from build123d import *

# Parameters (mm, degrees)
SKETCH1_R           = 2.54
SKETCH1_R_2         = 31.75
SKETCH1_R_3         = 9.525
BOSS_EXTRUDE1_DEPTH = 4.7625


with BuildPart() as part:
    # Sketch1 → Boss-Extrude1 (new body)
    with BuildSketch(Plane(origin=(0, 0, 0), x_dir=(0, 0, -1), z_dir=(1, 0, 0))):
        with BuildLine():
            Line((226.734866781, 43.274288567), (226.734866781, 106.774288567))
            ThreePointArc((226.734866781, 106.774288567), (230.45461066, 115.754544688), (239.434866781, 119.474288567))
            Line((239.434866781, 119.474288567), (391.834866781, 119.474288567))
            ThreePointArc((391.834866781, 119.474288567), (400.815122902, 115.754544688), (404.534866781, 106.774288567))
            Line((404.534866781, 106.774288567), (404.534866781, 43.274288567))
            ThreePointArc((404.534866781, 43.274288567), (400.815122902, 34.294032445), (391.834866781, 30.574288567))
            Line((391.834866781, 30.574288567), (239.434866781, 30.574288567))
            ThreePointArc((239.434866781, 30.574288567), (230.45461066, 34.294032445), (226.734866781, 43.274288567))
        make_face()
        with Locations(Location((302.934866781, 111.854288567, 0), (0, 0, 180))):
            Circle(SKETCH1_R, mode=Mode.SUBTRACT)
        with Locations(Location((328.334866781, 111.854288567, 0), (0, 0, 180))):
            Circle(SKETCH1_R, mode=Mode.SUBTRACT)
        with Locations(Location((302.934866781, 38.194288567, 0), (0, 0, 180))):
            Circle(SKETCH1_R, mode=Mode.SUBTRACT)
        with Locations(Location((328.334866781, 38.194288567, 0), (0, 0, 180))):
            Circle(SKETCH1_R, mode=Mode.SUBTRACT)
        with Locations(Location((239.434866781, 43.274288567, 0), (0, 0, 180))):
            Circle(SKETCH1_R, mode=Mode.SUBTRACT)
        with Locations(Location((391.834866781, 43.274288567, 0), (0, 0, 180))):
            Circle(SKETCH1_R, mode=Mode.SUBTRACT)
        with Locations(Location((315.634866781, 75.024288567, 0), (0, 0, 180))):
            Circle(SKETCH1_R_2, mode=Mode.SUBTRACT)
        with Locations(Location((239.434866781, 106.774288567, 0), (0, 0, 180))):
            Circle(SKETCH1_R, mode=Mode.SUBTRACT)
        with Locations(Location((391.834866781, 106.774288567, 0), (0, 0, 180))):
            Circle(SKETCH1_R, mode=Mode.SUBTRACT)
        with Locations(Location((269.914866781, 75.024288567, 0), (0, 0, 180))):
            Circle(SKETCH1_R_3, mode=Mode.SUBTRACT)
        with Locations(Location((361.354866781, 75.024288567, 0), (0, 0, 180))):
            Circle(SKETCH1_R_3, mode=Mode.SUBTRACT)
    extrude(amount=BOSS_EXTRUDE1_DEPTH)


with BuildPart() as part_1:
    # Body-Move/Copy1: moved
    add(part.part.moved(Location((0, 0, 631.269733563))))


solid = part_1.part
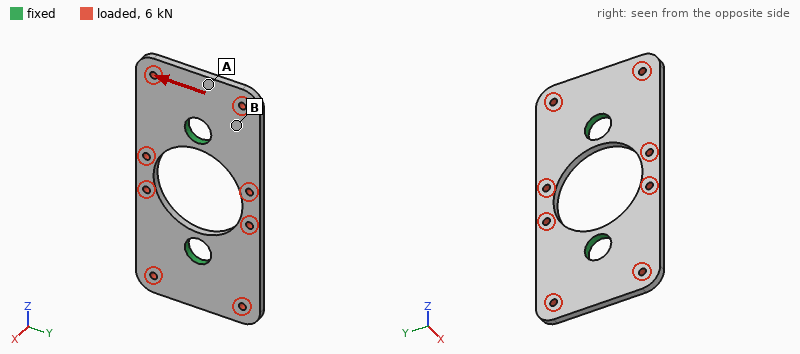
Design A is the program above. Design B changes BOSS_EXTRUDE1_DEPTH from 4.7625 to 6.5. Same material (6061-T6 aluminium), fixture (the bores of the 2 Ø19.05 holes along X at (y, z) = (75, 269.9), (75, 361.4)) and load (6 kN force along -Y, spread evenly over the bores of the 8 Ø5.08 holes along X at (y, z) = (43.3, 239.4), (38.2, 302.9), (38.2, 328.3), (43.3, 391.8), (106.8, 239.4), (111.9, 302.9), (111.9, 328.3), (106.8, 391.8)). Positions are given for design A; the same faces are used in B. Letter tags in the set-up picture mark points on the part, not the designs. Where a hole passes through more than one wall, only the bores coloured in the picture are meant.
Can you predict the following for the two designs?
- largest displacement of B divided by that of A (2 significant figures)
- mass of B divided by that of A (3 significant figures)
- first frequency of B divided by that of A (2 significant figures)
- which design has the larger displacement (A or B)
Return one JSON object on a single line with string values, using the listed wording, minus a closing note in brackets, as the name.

{"largest displacement of B divided by that of A": "0.73", "mass of B divided by that of A": "1.36", "first frequency of B divided by that of A": "1.3", "which design has the larger displacement": "A"}
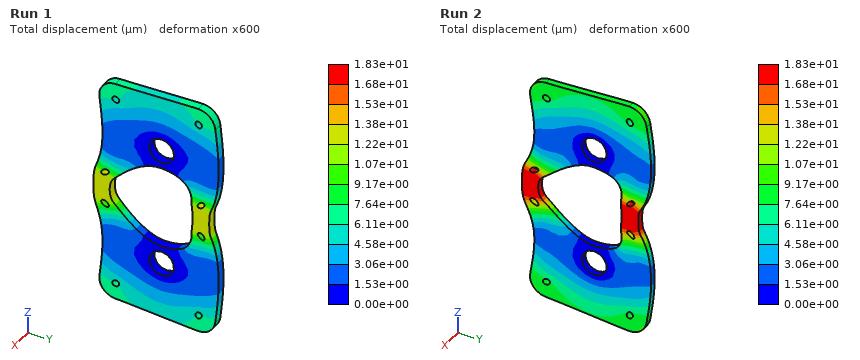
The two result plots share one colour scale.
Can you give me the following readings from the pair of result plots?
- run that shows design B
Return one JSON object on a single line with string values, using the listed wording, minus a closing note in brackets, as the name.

{"run that shows design B": "Run 1"}
